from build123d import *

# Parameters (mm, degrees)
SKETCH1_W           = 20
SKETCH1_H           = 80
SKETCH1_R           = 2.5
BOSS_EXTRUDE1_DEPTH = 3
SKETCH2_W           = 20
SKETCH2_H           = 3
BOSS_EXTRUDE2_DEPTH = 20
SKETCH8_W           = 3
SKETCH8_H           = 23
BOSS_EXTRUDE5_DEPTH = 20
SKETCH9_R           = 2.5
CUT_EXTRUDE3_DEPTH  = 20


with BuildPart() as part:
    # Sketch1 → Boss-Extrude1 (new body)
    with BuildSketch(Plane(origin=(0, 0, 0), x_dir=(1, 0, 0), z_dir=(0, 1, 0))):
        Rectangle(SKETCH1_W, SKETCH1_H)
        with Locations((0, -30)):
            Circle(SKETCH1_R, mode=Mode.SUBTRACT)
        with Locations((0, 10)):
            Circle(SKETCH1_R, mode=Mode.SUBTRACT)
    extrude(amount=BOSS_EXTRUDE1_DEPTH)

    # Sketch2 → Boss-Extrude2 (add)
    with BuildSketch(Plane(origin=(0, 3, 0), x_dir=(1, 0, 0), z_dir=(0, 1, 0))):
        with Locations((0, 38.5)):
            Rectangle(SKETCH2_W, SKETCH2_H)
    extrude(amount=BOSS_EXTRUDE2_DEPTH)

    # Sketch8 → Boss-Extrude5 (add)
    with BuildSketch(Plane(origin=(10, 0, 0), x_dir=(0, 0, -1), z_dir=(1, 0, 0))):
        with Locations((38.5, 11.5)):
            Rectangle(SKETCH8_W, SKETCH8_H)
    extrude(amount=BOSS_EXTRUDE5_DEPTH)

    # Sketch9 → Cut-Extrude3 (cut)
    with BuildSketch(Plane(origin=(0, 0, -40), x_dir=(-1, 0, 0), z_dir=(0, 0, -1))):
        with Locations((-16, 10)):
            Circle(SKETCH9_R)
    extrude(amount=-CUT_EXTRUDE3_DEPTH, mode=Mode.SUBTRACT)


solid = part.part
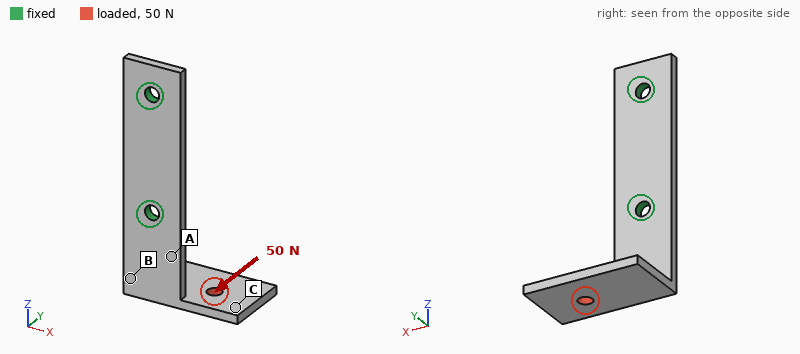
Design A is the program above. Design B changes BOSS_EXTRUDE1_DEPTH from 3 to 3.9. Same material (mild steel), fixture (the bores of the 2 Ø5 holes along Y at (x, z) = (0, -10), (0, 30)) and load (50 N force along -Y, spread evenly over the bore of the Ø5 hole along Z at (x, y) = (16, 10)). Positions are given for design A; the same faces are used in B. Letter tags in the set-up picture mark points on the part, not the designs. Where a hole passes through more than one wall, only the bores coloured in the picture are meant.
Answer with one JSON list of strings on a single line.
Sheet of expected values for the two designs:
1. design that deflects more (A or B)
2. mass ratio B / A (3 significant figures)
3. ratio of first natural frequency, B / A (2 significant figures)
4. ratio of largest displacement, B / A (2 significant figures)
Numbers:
["A", "1.19", "1.4", "0.48"]
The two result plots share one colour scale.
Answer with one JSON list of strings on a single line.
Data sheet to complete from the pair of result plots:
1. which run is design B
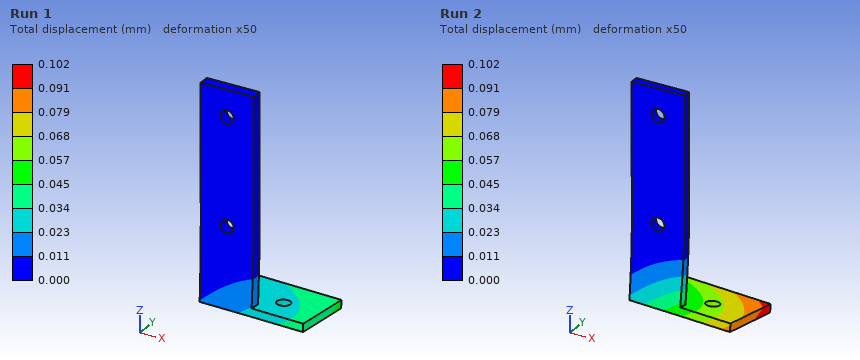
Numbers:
["Run 1"]
